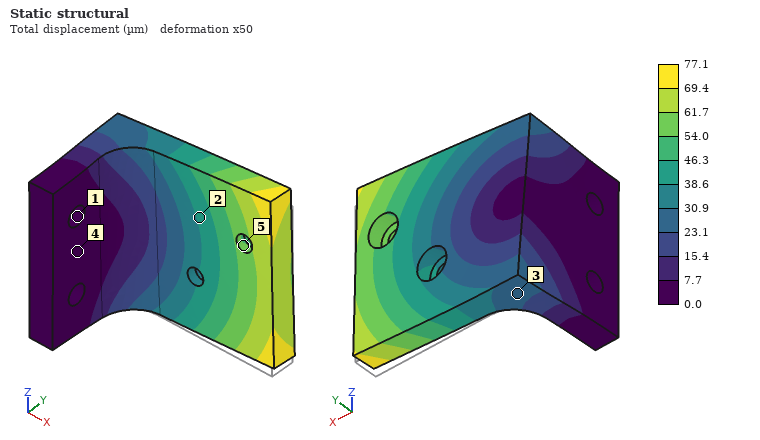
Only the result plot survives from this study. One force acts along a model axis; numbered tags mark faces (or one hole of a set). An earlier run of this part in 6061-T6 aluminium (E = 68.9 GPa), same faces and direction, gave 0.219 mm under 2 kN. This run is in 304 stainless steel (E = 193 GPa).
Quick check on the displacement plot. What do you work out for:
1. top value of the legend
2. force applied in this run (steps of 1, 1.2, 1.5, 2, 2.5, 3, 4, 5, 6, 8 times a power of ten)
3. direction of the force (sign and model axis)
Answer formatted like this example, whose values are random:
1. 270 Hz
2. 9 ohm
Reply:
1. 77.1 µm
2. 2 kN
3. +Z
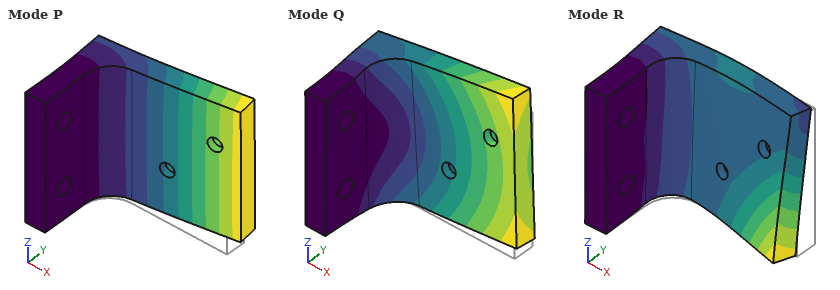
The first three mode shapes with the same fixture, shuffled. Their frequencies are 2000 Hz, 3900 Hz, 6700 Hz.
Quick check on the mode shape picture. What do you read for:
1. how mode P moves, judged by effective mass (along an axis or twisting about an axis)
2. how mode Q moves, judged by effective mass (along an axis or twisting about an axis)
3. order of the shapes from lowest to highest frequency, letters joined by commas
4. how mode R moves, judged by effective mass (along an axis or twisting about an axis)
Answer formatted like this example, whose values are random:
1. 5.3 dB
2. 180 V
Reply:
1. along Y
2. along Z
3. P, Q, R
4. along X
